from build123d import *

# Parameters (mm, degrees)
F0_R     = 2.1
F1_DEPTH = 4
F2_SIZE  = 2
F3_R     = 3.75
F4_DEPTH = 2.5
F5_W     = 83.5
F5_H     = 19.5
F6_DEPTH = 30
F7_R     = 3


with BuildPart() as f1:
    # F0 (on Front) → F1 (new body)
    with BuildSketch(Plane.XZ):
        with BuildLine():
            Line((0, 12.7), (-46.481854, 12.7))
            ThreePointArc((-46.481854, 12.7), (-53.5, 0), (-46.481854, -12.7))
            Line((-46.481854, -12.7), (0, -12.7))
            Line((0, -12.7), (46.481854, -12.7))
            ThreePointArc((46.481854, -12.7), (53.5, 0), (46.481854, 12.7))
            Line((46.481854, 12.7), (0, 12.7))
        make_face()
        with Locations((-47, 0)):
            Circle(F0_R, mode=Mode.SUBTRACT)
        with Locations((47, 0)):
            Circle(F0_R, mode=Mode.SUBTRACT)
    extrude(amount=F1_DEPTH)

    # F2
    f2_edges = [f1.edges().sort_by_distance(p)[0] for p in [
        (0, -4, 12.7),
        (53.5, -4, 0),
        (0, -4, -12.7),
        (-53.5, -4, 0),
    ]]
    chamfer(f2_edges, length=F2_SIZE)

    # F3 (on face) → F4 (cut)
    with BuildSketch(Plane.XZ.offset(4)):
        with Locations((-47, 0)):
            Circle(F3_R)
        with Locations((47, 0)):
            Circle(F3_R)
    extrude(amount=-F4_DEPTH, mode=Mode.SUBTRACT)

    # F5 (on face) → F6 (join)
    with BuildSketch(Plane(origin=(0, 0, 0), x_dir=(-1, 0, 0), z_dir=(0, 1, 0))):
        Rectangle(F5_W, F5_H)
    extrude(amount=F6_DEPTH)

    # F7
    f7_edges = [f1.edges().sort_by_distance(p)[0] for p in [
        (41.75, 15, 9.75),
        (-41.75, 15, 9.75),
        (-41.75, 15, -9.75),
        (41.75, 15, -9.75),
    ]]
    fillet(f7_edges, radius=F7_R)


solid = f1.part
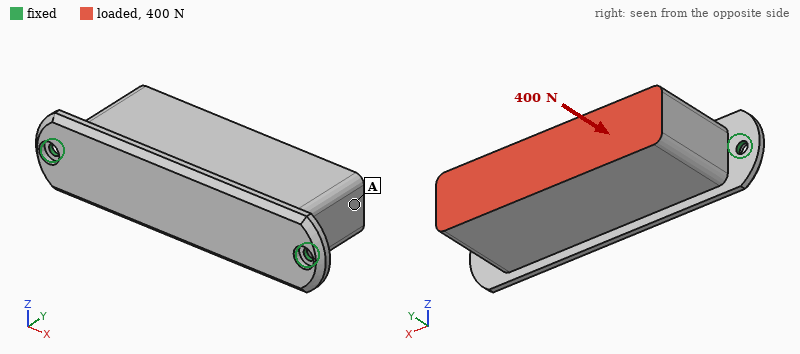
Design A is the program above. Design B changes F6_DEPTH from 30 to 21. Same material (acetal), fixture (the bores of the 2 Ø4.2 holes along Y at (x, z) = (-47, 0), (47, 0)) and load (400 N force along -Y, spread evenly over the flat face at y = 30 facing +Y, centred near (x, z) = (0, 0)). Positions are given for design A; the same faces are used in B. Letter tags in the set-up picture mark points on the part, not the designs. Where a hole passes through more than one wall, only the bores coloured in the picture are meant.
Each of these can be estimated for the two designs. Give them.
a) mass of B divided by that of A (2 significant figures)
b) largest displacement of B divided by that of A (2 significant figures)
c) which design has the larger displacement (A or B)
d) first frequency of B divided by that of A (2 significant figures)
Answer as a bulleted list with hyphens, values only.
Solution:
- 0.75
- 1.2
- B
- 1.6
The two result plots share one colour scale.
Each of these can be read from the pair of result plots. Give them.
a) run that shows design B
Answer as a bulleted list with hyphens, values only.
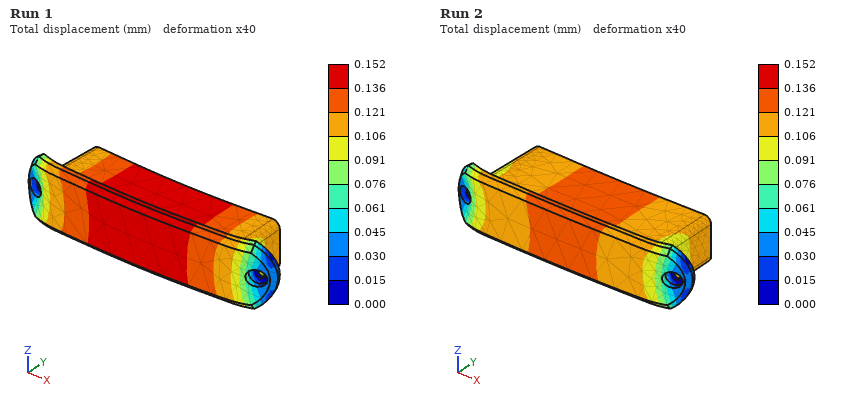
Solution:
- Run 1
